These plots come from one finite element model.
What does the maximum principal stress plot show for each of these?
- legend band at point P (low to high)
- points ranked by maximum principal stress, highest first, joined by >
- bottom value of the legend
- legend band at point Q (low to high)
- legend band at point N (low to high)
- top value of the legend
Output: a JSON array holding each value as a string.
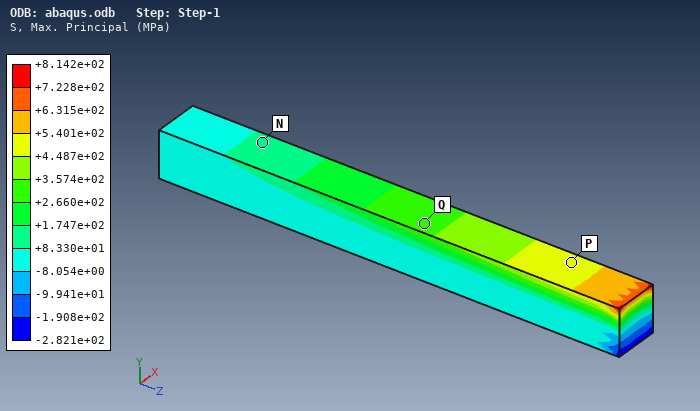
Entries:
["+4.487e+02 to +5.401e+02 MPa", "P > Q > N", "-2.821e+02 MPa", "+2.660e+02 to +3.574e+02 MPa", "+8.330e+01 to +1.747e+02 MPa", "+8.142e+02 MPa"]
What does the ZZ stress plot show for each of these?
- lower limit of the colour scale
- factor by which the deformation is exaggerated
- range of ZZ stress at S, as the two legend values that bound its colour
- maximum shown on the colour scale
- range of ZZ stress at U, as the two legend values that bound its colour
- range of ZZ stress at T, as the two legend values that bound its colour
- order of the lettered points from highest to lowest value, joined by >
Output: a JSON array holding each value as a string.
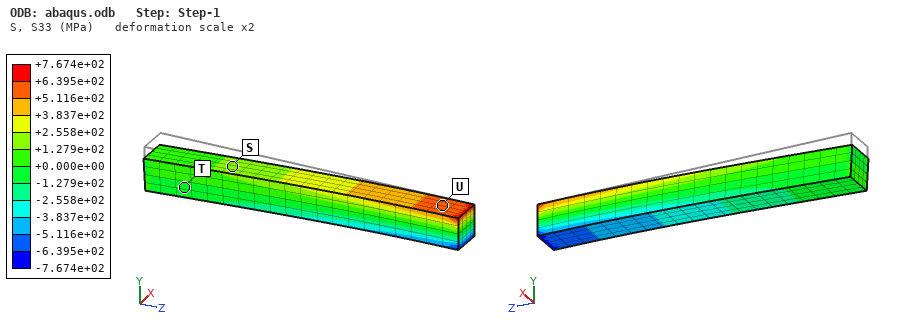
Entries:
["-7.674e+02 MPa", "2", "+1.279e+02 to +2.558e+02 MPa", "+7.674e+02 MPa", "+5.116e+02 to +6.395e+02 MPa", "-1.279e+02 to +0.000e+00 MPa", "U > S > T"]
